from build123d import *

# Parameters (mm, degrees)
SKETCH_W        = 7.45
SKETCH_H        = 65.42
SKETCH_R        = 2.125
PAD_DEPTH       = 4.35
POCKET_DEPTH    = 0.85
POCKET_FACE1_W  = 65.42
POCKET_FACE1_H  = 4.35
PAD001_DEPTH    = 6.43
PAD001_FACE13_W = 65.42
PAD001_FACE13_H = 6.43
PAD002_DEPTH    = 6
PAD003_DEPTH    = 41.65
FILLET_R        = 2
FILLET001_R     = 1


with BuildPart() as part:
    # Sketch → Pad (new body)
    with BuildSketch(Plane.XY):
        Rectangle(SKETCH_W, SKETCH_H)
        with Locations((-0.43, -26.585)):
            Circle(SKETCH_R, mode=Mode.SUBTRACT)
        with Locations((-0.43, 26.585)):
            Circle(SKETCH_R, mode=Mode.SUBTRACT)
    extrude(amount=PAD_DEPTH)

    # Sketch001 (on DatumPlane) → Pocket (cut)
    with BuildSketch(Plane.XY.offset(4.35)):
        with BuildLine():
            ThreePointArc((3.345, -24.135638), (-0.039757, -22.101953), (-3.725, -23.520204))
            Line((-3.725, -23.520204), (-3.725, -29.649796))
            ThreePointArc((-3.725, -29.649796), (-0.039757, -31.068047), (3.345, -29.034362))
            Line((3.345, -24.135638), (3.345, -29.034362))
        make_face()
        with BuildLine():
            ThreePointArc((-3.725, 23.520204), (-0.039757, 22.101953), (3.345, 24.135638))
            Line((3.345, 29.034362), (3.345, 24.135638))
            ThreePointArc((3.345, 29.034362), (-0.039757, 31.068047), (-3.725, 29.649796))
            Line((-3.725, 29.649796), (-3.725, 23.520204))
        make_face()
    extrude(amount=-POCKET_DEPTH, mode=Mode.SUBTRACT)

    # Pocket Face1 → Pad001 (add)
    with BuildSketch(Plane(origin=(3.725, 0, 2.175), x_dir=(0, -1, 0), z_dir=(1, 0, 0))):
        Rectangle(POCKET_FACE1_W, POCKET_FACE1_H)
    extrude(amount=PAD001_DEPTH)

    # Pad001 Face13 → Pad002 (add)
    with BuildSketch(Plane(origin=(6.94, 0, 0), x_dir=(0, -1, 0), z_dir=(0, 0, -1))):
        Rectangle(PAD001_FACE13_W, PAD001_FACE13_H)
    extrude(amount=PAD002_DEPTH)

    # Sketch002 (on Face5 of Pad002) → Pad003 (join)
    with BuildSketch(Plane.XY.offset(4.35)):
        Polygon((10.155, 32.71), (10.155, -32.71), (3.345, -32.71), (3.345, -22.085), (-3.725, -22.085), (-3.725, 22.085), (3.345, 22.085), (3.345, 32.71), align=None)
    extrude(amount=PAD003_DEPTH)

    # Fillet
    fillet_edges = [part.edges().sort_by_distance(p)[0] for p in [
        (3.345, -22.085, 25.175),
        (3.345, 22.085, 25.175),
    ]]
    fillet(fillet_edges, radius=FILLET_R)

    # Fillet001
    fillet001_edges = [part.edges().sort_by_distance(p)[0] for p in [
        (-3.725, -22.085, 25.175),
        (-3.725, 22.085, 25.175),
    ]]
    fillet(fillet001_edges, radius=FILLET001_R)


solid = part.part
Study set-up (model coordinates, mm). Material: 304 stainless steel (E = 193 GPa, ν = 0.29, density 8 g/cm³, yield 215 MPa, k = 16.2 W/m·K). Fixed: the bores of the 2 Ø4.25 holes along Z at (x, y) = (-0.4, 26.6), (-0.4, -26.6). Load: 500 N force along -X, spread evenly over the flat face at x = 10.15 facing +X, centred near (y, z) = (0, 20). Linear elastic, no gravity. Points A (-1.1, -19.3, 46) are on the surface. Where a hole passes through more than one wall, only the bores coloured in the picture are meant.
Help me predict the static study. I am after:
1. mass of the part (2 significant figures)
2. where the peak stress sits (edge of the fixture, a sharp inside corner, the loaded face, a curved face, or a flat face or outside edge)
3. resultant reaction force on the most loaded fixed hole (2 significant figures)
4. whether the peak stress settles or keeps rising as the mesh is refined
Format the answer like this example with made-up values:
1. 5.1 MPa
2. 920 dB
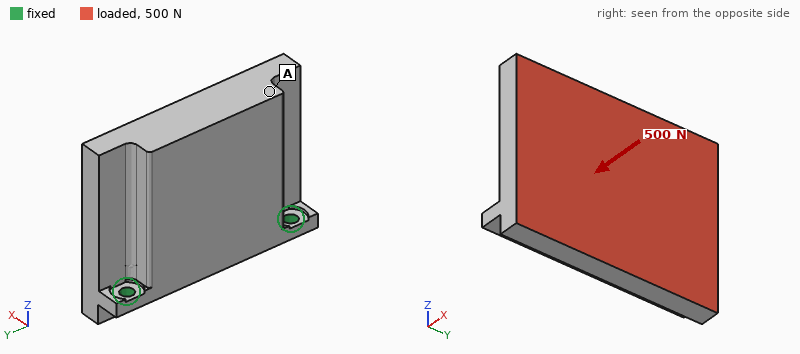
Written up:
1. 300 g
2. edge of the fixture
3. 320 N
4. keeps rising
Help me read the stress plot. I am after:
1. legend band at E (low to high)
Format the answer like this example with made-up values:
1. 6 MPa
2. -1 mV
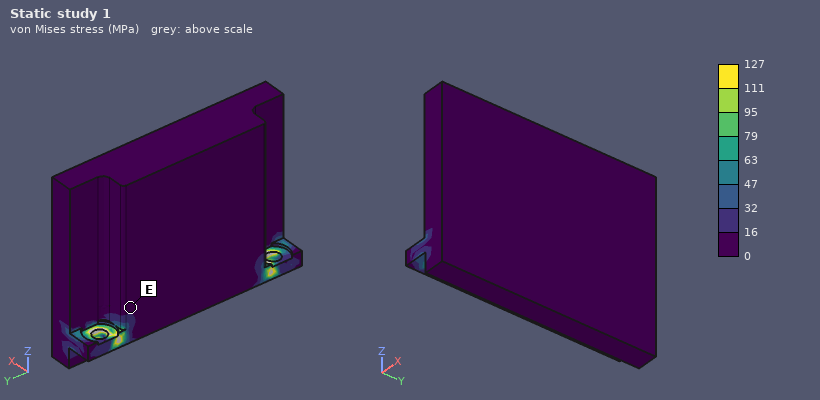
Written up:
1. 0 to 16 MPa
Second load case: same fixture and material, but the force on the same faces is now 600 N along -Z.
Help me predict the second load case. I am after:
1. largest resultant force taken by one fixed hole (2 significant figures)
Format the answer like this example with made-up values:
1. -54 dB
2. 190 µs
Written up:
1. 300 N
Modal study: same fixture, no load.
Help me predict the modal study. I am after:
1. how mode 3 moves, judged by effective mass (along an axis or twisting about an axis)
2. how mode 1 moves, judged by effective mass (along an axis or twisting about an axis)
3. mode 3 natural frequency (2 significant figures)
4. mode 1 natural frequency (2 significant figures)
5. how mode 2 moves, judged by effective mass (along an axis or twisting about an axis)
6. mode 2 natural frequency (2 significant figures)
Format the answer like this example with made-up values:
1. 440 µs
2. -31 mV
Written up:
1. along Y
2. along X
3. 7400 Hz
4. 1100 Hz
5. along Y
6. 6300 Hz
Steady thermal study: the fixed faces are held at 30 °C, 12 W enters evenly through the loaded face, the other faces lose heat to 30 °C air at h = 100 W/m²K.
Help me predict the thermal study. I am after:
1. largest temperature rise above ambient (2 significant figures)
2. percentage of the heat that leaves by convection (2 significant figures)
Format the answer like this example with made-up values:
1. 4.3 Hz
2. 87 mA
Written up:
1. 17 K
2. 69 %
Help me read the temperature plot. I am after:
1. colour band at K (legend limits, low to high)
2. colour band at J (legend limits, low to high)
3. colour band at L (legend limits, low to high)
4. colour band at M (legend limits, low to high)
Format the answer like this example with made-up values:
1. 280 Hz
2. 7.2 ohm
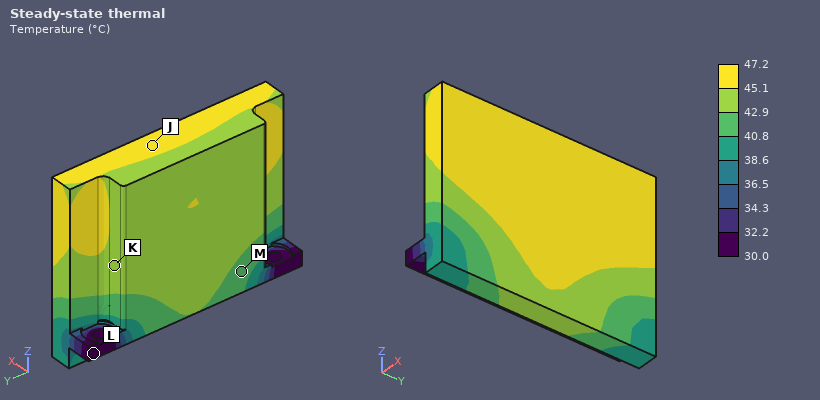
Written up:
1. 42.9 to 45.1 °C
2. 45.1 to 47.2 °C
3. 30.0 to 32.2 °C
4. 40.8 to 42.9 °C
